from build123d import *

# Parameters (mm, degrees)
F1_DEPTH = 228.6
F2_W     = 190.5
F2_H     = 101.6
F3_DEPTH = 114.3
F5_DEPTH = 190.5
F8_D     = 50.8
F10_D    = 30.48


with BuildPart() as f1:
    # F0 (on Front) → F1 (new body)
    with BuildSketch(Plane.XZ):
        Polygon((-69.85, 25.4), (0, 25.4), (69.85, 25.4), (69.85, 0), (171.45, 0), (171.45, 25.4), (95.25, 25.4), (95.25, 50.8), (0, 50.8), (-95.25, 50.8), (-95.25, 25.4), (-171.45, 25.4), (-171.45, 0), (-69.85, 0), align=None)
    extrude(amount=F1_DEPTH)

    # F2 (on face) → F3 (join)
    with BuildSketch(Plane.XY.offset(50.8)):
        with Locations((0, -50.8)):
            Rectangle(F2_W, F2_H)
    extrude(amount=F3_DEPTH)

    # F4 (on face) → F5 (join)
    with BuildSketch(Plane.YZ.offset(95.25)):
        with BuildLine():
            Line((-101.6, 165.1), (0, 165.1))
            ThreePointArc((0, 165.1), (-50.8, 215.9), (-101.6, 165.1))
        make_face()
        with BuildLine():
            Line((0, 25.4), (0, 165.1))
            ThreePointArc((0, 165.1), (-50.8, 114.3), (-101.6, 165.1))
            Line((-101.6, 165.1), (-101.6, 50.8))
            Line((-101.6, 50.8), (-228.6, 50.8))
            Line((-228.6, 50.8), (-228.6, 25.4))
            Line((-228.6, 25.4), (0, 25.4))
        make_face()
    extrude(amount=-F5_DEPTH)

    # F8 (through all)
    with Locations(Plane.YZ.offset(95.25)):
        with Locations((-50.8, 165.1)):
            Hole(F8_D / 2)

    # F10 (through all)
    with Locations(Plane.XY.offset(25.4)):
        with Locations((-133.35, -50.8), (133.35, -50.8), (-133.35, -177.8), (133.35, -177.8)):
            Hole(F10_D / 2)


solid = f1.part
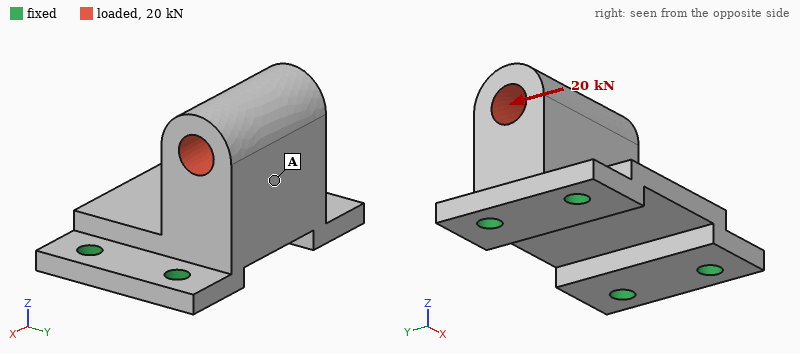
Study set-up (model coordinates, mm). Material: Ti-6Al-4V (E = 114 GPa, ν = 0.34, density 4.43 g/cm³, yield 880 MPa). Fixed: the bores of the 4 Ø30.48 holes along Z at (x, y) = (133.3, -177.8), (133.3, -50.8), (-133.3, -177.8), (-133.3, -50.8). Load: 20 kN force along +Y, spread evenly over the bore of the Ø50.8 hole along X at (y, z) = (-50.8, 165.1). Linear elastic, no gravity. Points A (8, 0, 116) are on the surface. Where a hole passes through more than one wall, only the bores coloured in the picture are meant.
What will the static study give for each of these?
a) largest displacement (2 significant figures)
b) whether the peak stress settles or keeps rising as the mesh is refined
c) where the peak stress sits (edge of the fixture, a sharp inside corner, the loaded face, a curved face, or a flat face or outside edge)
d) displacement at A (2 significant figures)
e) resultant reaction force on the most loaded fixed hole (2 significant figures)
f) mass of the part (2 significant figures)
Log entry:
0.12 mm
keeps rising
edge of the fixture
0.069 mm
18 kN
21 kg
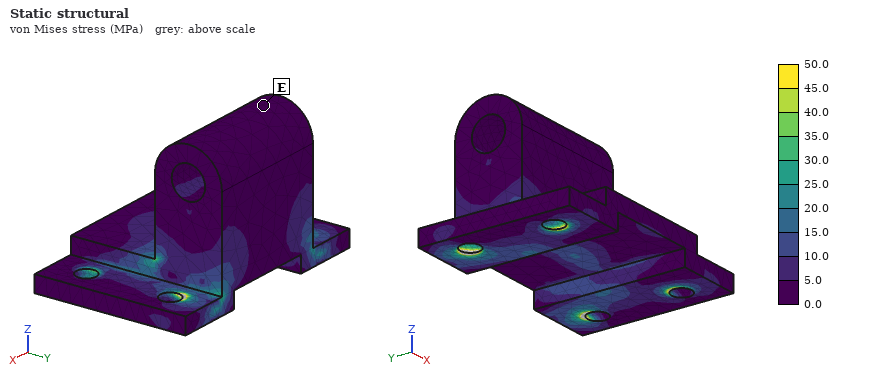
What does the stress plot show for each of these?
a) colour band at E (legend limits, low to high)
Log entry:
0.0 to 5.0 MPa
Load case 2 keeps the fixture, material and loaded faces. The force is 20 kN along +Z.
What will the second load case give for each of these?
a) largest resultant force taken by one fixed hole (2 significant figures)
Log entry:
11 kN
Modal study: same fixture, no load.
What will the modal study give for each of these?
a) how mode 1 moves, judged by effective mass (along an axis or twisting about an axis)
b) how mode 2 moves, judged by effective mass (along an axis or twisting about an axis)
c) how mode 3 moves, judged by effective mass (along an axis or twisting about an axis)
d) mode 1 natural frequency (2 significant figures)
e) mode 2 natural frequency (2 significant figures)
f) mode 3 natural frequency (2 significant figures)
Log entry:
along Y
along X
along Z
860 Hz
1600 Hz
1900 Hz
